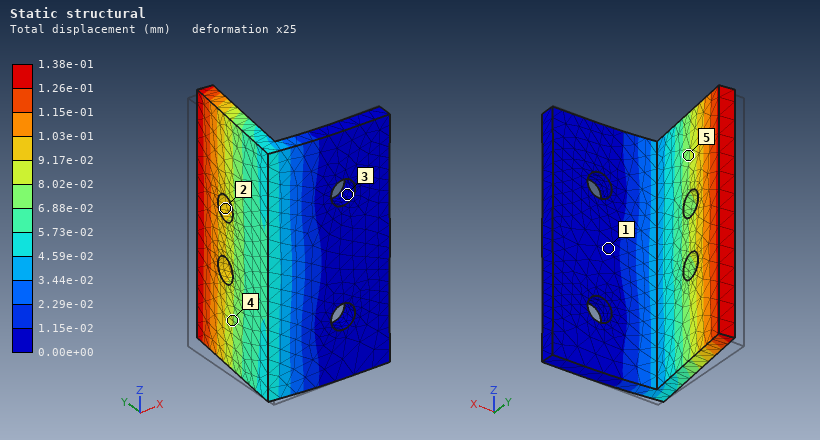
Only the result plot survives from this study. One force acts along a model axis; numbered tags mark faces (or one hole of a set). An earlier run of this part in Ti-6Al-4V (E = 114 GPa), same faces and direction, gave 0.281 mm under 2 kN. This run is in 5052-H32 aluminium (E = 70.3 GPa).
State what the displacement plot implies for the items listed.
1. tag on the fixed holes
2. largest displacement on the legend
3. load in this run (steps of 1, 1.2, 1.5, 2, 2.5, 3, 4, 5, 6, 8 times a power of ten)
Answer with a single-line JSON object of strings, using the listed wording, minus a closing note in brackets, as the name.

{"tag on the fixed holes": "3", "largest displacement on the legend": "1.38e-01 mm", "load in this run": "600 N"}
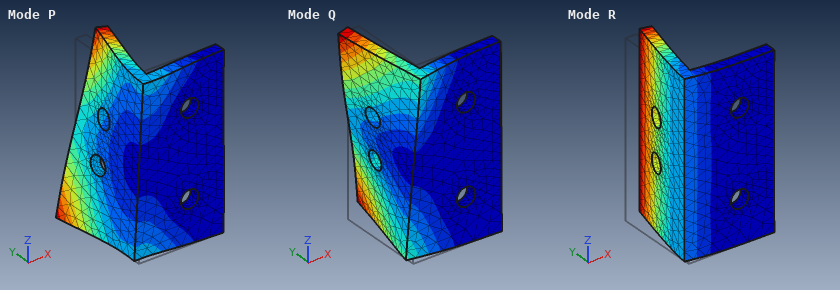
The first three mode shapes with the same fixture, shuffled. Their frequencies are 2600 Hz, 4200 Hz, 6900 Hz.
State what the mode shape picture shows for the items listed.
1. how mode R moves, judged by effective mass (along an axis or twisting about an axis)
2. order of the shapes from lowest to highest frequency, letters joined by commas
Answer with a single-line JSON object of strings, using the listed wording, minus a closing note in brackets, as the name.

{"how mode R moves, judged by effective mass": "along X", "order of the shapes from lowest to highest frequency, letters joined by commas": "R, Q, P"}
